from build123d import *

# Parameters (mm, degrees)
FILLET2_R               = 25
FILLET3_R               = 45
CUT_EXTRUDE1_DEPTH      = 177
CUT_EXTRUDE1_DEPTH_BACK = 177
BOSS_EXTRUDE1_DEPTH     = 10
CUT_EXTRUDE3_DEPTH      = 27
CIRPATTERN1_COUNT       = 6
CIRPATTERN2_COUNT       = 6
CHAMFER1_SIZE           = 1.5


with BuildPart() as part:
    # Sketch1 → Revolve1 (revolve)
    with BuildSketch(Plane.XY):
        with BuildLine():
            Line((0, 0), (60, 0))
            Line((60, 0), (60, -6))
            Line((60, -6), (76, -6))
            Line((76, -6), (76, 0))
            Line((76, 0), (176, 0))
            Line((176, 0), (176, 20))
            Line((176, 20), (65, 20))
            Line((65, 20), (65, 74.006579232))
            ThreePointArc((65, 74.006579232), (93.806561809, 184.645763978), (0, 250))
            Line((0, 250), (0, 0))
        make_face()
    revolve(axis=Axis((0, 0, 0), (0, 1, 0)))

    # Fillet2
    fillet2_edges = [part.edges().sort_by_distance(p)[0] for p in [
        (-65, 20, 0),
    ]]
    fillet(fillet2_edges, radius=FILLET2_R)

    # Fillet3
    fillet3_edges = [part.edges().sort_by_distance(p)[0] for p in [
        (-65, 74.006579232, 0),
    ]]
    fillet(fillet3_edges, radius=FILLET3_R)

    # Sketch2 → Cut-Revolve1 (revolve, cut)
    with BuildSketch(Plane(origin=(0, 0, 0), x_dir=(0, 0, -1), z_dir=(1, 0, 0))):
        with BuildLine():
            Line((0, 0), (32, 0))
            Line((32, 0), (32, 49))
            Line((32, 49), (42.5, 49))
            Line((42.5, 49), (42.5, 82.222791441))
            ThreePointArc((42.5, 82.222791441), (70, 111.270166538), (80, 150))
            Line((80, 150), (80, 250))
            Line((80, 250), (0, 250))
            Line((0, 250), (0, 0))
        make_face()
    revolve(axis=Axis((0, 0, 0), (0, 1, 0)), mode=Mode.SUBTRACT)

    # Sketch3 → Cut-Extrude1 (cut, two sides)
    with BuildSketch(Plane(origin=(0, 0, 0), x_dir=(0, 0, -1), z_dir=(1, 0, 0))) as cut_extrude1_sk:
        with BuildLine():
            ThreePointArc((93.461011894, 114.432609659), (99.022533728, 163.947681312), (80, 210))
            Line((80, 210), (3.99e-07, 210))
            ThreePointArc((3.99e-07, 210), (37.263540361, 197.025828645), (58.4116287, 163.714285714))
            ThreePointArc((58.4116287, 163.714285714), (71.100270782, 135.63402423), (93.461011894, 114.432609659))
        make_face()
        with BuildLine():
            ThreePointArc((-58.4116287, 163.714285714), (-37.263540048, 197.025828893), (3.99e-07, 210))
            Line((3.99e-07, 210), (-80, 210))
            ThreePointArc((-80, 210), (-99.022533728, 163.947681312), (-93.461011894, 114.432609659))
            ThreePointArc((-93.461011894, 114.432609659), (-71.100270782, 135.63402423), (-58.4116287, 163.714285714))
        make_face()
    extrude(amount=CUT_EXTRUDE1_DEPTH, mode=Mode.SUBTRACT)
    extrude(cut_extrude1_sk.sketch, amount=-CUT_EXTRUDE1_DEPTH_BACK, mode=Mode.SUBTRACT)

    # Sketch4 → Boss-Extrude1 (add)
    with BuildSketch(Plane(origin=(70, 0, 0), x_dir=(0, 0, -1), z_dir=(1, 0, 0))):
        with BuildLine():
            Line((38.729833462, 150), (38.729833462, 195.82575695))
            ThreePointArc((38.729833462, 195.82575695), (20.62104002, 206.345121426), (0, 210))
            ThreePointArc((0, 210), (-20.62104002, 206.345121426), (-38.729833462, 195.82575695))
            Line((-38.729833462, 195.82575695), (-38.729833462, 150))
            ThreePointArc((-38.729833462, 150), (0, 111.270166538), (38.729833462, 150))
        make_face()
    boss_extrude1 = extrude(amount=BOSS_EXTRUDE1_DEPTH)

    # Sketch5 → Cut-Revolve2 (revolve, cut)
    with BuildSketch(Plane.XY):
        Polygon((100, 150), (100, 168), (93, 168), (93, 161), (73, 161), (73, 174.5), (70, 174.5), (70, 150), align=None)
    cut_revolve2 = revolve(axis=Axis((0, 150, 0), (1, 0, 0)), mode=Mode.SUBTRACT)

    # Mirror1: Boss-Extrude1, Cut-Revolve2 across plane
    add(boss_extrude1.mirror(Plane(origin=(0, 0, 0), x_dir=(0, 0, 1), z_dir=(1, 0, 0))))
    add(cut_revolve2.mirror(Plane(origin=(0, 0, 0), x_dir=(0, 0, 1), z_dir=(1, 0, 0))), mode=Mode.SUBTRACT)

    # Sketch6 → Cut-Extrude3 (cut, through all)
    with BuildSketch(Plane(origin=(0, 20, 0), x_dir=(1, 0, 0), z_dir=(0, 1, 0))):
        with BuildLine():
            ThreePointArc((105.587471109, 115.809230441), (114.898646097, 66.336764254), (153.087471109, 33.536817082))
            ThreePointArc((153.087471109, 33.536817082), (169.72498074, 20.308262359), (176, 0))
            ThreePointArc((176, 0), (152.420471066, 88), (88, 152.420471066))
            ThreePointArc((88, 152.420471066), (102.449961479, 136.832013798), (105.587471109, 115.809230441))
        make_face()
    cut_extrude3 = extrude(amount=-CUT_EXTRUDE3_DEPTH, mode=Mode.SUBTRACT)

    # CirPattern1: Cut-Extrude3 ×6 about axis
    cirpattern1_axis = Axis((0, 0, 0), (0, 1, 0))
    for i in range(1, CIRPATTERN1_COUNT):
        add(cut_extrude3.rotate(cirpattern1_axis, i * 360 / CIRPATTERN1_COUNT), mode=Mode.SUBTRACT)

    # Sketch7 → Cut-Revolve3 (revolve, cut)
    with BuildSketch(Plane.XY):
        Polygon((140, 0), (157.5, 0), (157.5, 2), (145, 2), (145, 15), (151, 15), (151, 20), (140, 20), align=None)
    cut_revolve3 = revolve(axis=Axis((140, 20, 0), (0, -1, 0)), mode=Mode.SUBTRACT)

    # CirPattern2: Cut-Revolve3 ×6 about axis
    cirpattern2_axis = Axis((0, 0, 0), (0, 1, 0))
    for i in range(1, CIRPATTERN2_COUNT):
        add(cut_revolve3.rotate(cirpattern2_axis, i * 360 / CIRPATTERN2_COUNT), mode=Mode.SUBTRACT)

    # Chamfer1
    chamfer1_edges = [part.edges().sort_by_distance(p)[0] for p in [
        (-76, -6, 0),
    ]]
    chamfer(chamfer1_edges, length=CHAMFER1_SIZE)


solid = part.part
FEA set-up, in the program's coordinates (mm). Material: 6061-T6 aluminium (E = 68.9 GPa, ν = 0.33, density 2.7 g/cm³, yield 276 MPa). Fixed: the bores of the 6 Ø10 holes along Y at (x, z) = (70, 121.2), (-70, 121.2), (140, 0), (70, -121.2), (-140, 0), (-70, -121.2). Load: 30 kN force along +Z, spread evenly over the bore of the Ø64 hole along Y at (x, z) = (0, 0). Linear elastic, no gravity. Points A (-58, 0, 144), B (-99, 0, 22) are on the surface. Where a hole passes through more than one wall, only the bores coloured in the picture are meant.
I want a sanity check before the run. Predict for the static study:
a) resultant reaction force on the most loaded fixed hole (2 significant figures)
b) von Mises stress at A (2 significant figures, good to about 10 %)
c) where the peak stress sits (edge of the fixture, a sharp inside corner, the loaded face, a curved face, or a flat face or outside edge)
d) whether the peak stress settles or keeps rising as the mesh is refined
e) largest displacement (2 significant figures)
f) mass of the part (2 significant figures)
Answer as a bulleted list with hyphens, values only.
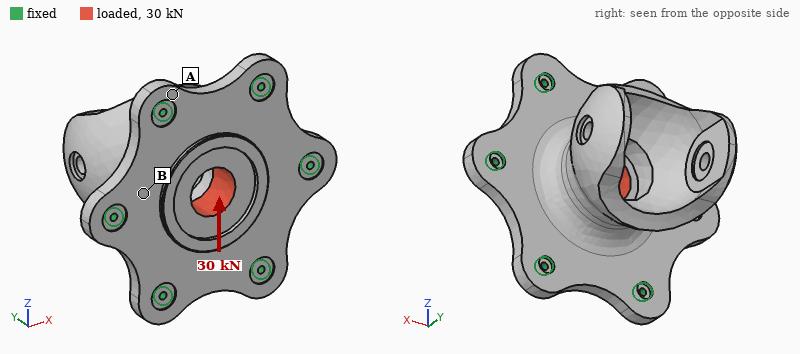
- 6.9 kN
- 4.0 MPa
- edge of the fixture
- keeps rising
- 29 µm
- 7.9 kg
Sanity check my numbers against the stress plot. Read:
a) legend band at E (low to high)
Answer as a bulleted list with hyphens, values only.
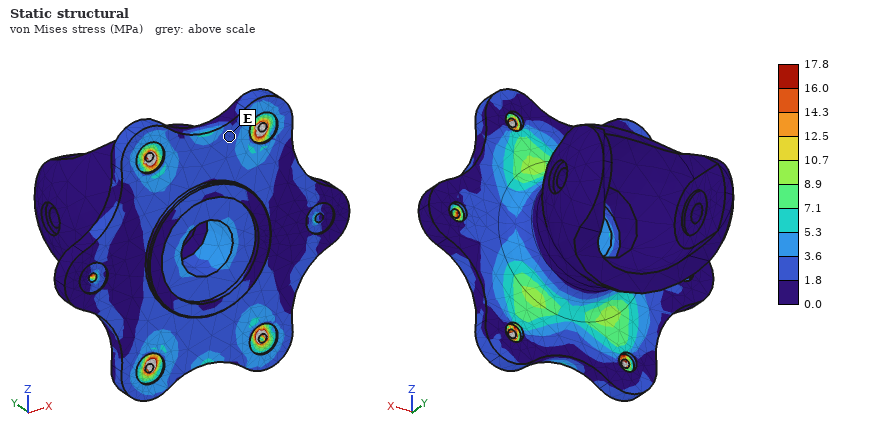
- 1.8 to 3.6 MPa
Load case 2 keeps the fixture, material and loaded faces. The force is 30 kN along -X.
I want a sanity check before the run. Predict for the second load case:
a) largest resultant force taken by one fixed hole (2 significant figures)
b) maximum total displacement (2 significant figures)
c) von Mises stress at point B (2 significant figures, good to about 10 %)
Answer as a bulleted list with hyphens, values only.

- 7.9 kN
- 30 µm
- 3.4 MPa
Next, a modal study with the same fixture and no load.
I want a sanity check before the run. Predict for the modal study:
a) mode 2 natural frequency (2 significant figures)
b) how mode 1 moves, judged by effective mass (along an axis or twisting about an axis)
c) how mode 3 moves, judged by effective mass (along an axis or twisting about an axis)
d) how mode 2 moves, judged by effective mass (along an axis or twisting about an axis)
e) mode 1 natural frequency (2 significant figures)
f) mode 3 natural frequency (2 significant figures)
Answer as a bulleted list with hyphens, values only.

- 1100 Hz
- along X
- along Y
- along Z
- 990 Hz
- 1200 Hz
